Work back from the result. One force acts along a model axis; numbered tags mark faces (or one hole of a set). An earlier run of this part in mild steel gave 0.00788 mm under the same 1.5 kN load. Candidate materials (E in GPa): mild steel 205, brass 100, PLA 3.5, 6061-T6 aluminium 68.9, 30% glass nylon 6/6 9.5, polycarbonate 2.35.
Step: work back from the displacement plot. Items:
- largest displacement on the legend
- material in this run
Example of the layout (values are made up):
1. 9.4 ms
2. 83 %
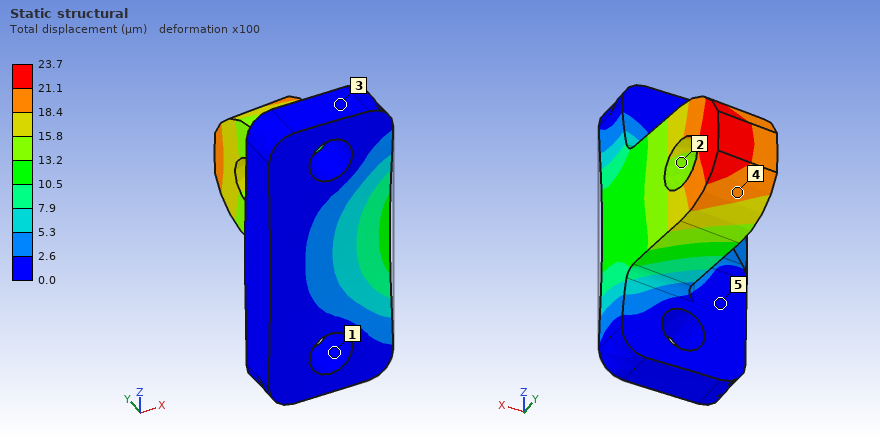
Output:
1. 23.7 µm
2. 6061-T6 aluminium
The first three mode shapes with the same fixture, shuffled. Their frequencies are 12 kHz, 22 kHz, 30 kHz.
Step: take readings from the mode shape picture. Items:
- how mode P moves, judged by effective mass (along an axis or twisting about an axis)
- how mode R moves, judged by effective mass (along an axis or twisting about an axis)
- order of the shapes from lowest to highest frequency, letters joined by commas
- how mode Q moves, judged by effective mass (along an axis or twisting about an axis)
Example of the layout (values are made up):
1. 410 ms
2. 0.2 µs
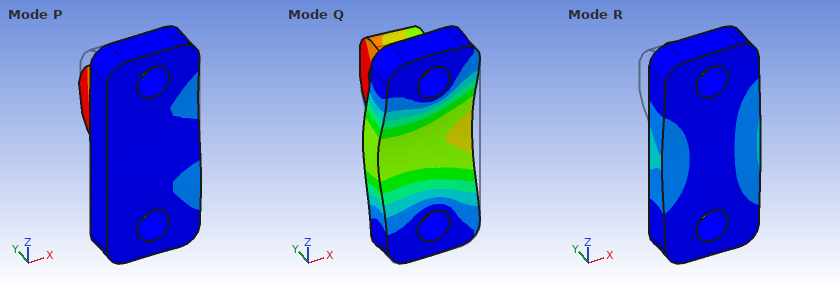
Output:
1. along Z
2. along X
3. R, P, Q
4. along Y
